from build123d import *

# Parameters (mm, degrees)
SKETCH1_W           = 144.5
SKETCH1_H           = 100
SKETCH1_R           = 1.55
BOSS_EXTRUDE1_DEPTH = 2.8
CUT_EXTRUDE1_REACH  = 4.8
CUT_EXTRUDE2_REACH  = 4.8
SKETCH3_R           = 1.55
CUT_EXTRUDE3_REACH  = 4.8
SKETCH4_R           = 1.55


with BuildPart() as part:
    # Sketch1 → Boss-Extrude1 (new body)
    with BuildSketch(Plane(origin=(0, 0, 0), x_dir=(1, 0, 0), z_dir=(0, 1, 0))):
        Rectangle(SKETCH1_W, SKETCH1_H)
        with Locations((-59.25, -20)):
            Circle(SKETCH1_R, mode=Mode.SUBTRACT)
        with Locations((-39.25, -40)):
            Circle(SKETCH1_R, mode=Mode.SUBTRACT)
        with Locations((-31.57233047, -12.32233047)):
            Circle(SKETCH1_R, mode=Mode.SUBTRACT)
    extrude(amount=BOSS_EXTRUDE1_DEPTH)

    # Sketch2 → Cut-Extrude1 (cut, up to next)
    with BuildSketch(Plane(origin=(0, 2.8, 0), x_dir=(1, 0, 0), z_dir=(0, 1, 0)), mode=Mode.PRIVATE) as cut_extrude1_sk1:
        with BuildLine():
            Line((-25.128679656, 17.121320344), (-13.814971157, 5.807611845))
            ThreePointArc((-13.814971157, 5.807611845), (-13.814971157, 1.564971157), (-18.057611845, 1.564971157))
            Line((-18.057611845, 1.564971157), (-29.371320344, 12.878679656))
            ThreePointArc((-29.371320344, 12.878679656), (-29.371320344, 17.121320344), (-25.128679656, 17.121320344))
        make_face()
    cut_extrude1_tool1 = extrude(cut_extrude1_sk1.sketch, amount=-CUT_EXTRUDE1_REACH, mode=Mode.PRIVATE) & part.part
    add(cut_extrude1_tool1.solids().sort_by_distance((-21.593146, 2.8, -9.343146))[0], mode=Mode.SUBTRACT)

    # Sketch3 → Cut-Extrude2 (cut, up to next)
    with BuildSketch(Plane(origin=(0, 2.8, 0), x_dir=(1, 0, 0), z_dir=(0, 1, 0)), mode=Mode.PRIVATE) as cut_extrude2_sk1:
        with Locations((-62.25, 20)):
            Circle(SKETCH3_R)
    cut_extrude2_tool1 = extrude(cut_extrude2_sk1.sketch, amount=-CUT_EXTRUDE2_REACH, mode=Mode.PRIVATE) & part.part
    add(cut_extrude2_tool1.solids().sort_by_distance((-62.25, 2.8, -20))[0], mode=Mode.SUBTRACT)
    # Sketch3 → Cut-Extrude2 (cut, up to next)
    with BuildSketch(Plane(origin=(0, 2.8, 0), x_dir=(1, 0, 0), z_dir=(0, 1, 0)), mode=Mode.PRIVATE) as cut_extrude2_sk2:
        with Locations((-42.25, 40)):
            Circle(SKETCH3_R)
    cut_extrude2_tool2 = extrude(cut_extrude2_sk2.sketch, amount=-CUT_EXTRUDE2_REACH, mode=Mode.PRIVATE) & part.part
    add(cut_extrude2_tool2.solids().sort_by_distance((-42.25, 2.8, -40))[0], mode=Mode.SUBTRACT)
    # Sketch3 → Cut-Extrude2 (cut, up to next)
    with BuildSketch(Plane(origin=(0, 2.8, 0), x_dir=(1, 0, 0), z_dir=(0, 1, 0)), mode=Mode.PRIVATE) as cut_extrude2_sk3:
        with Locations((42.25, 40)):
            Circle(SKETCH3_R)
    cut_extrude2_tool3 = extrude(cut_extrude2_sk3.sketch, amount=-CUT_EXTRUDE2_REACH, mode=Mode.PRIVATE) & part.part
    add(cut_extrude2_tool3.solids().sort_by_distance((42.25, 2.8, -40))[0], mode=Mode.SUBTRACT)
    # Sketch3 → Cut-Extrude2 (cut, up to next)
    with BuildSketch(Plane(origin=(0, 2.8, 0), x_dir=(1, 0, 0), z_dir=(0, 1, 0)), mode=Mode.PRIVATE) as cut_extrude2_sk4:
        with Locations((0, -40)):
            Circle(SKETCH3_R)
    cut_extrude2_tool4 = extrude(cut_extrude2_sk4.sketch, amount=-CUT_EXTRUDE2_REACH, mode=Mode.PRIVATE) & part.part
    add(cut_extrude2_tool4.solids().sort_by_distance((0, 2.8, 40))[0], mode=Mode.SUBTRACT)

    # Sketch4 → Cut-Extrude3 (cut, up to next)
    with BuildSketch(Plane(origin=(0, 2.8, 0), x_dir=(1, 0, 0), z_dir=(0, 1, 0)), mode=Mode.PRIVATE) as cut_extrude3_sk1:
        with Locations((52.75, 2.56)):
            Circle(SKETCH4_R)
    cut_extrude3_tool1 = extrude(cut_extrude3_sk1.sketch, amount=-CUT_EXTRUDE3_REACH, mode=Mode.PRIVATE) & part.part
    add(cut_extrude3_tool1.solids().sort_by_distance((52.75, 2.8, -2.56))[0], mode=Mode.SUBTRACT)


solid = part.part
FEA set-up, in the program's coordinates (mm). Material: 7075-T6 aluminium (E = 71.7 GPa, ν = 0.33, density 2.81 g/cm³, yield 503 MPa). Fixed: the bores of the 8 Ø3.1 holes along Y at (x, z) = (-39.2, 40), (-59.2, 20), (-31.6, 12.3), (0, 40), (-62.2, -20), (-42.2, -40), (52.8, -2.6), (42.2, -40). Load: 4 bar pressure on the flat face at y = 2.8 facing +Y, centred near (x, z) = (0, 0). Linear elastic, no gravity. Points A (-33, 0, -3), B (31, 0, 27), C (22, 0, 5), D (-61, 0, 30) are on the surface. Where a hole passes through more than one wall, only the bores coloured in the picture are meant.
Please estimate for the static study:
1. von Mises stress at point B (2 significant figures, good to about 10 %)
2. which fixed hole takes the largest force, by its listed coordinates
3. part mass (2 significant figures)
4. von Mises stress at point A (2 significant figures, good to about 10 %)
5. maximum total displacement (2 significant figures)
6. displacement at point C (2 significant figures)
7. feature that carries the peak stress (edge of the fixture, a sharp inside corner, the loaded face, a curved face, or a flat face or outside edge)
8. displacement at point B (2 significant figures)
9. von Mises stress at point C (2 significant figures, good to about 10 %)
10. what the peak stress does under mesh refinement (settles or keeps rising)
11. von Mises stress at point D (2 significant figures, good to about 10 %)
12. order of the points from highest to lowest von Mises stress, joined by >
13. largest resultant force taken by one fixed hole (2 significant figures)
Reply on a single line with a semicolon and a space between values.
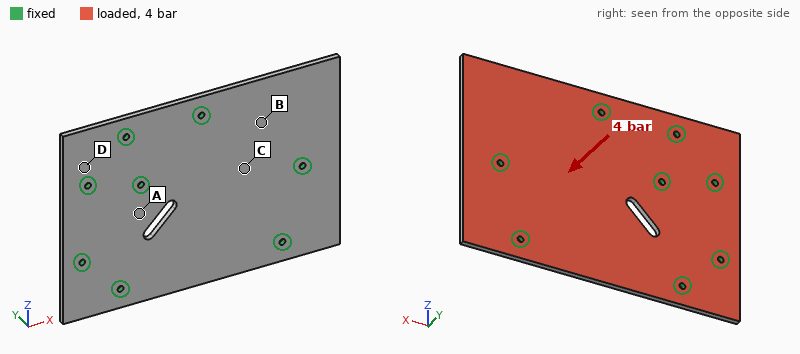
120 MPa; (52.8, -2.6); 110 g; 51 MPa; 1.7 mm; 0.29 mm; edge of the fixture; 0.46 mm; 85 MPa; keeps rising; 23 MPa; B > C > A > D; 1.4 kN
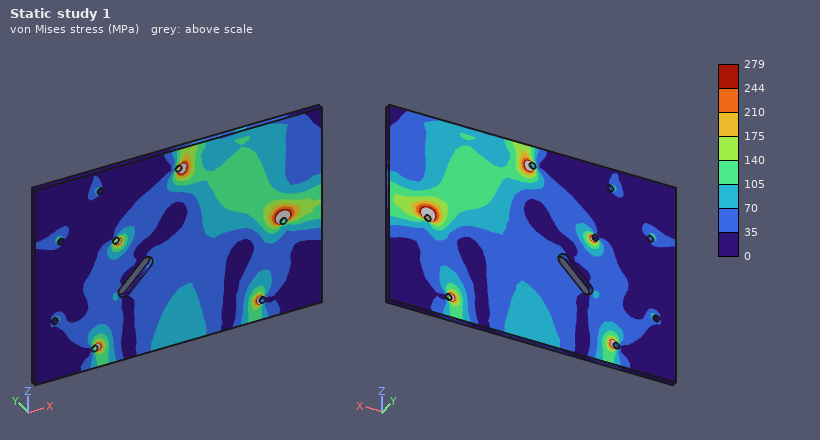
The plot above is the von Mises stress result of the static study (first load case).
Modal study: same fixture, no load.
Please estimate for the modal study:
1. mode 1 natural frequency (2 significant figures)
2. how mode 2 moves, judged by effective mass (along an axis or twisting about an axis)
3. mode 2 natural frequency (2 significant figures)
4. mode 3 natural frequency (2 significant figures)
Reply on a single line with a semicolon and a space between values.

1200 Hz; along Y; 2000 Hz; 2800 Hz
